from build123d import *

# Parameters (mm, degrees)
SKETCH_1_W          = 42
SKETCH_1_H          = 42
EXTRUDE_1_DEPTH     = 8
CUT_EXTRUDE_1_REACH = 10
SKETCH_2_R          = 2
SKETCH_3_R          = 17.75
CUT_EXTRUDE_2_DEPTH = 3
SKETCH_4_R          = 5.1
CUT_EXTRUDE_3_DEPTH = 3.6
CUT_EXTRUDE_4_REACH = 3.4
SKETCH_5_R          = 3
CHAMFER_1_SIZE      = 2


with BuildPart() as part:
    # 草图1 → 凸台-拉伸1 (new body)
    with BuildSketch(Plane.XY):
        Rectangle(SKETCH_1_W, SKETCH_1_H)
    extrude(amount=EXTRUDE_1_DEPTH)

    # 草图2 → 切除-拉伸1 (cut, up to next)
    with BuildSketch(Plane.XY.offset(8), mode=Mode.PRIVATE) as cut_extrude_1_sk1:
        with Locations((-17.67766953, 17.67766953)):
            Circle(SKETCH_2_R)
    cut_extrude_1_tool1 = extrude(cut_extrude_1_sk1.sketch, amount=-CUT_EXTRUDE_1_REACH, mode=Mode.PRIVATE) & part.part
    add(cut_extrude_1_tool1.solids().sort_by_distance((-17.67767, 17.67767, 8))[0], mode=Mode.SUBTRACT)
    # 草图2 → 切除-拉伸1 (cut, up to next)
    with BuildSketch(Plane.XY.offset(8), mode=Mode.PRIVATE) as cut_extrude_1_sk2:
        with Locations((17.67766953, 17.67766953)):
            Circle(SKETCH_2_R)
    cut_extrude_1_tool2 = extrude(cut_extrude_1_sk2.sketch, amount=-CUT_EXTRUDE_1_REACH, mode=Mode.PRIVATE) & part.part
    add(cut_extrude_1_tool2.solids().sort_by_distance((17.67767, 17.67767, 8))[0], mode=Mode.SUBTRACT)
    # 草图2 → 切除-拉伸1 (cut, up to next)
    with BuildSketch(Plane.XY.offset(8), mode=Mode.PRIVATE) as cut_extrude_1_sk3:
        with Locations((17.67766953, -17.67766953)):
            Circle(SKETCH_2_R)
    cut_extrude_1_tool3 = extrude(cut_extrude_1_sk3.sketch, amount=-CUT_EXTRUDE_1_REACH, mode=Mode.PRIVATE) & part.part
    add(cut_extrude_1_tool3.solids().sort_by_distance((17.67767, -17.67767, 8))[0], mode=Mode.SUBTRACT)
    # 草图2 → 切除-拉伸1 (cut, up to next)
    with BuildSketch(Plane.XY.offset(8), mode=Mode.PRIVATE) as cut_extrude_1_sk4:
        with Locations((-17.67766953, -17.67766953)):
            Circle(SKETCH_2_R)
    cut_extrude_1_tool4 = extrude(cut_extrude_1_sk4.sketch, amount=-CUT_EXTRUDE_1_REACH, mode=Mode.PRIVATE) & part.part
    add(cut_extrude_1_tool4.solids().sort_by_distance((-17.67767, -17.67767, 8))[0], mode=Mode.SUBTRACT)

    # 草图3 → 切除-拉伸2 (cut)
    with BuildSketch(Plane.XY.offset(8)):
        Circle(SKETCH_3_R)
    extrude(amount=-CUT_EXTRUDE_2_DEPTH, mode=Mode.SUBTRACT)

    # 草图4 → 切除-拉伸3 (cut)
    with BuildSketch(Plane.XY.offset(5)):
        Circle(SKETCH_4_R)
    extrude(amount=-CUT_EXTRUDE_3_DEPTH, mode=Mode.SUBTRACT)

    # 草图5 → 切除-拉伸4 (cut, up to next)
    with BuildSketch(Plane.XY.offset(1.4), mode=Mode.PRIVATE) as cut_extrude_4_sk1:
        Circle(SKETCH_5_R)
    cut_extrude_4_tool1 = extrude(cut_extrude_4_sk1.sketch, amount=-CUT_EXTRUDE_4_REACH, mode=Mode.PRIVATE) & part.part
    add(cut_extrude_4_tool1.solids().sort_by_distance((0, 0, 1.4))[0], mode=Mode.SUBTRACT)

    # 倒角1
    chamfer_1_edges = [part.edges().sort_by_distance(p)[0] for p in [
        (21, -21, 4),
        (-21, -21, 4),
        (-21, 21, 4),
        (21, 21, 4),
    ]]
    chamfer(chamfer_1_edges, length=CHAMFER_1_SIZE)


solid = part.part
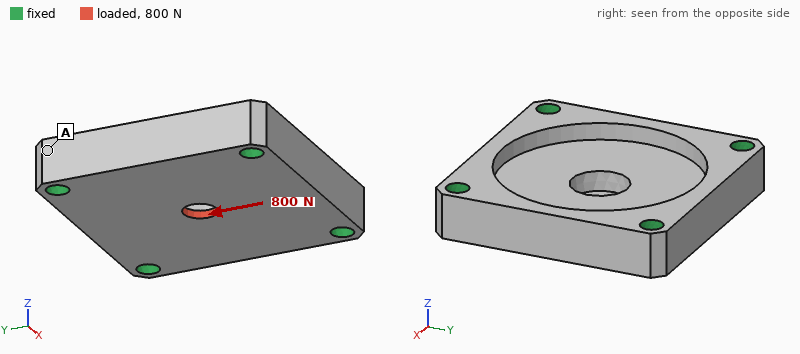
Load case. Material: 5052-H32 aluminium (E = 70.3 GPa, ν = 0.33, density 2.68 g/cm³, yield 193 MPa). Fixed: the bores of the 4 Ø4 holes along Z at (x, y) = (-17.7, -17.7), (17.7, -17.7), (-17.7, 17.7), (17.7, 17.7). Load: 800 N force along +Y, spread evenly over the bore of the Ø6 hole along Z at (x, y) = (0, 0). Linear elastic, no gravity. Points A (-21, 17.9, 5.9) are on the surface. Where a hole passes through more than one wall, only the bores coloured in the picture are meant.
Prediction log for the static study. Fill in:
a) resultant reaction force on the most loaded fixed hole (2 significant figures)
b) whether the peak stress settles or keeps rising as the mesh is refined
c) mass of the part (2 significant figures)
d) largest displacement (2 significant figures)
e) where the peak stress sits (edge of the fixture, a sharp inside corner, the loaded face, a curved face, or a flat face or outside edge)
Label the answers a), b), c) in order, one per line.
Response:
a) 230 N
b) keeps rising
c) 28 g
d) 3.6 µm
e) a sharp inside corner
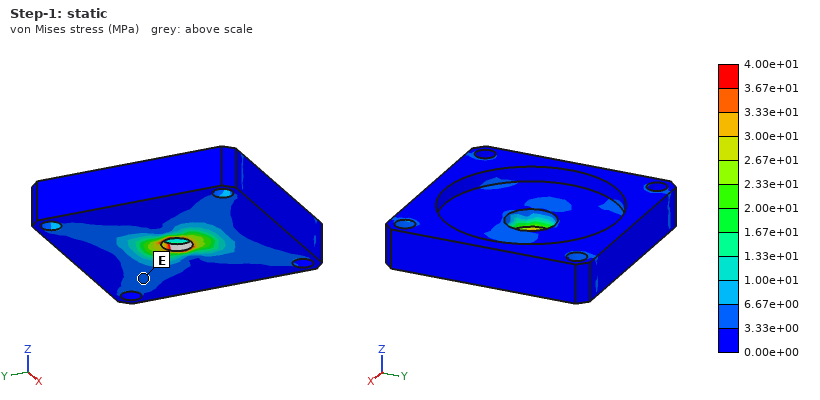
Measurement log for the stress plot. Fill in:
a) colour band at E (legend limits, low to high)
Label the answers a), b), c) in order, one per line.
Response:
a) 3.33e+00 to 6.67e+00 MPa
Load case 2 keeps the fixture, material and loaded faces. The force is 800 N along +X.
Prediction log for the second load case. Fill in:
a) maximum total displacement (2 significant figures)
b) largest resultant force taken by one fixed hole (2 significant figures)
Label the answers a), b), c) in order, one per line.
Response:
a) 3.6 µm
b) 230 N
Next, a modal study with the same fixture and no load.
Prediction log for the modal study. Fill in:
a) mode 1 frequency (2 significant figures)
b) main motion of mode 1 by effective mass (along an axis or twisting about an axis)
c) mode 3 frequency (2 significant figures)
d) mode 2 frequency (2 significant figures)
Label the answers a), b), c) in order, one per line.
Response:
a) 19 kHz
b) along Z
c) 28 kHz
d) 28 kHz
